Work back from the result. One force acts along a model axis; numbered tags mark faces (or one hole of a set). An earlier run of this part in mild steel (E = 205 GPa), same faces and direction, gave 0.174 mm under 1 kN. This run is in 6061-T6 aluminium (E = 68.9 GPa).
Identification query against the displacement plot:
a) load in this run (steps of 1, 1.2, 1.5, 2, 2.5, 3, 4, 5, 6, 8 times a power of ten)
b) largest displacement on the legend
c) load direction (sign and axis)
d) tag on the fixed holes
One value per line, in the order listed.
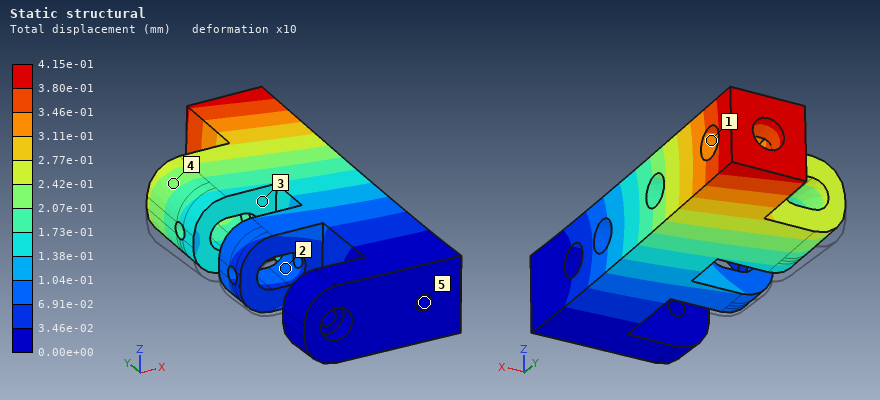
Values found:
800 N
4.15e-01 mm
+Z
5
